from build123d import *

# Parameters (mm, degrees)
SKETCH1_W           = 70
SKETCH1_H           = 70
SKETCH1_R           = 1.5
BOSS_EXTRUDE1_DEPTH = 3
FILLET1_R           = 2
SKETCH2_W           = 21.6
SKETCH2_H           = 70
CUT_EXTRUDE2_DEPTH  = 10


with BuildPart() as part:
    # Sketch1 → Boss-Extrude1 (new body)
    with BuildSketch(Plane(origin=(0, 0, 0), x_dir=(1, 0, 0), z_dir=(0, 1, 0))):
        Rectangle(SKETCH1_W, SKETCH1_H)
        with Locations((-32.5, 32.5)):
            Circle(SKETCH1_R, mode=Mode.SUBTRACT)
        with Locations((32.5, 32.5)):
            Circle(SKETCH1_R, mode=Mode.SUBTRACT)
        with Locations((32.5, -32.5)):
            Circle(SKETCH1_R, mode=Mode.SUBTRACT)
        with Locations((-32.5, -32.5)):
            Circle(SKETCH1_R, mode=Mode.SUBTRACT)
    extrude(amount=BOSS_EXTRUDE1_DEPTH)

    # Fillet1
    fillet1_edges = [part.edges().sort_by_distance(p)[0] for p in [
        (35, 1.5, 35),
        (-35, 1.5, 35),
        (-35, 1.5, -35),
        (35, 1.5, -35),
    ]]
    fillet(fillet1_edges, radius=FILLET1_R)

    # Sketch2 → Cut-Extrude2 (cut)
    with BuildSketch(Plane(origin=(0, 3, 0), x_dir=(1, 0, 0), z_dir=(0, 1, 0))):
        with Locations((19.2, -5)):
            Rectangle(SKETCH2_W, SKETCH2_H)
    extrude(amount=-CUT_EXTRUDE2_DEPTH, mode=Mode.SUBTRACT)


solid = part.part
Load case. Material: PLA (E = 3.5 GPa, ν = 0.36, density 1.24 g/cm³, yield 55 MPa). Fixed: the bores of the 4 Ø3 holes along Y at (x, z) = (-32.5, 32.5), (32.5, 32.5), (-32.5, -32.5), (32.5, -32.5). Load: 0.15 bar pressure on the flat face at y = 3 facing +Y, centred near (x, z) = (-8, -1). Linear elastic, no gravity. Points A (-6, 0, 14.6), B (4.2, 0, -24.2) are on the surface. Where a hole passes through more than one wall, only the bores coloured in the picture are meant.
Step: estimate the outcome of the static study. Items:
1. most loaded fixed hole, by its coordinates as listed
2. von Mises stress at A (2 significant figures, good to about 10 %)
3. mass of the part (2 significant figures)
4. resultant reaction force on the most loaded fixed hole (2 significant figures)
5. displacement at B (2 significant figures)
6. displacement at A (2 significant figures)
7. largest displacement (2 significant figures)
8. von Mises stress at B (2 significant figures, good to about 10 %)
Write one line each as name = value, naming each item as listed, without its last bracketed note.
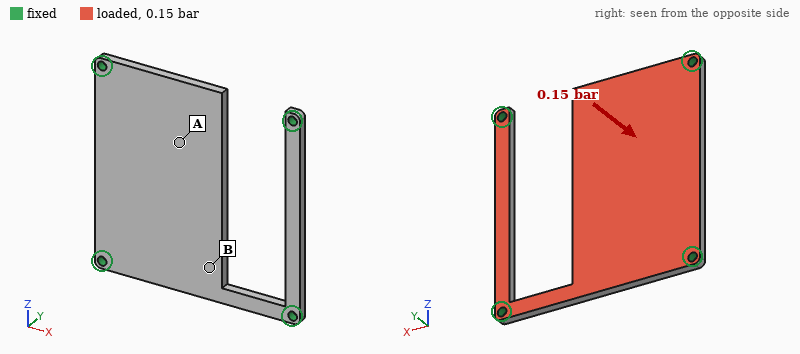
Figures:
most loaded fixed hole, by its coordinates as listed = (-32.5, 32.5)
von Mises stress at A = 2.9 MPa
mass of the part = 13 g
resultant reaction force on the most loaded fixed hole = 22 N
displacement at B = 0.45 mm
displacement at A = 0.64 mm
largest displacement = 1.0 mm
von Mises stress at B = 5.8 MPa
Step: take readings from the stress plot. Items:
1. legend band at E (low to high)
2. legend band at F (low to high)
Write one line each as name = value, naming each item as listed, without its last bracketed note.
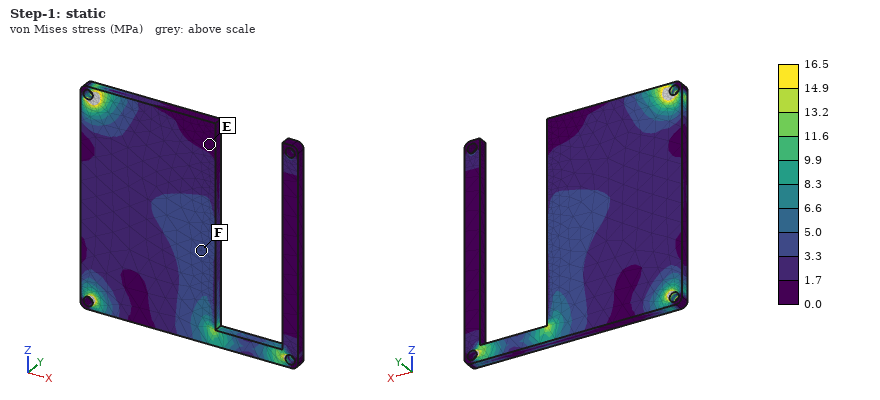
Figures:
legend band at E = 0.0 to 1.7 MPa
legend band at F = 3.3 to 5.0 MPa
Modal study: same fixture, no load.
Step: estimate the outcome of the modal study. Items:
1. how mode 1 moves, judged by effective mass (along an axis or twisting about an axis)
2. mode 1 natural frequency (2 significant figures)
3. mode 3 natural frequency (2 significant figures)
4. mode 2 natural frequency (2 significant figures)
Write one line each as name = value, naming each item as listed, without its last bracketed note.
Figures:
how mode 1 moves, judged by effective mass = along Y
mode 1 natural frequency = 420 Hz
mode 3 natural frequency = 1300 Hz
mode 2 natural frequency = 950 Hz
